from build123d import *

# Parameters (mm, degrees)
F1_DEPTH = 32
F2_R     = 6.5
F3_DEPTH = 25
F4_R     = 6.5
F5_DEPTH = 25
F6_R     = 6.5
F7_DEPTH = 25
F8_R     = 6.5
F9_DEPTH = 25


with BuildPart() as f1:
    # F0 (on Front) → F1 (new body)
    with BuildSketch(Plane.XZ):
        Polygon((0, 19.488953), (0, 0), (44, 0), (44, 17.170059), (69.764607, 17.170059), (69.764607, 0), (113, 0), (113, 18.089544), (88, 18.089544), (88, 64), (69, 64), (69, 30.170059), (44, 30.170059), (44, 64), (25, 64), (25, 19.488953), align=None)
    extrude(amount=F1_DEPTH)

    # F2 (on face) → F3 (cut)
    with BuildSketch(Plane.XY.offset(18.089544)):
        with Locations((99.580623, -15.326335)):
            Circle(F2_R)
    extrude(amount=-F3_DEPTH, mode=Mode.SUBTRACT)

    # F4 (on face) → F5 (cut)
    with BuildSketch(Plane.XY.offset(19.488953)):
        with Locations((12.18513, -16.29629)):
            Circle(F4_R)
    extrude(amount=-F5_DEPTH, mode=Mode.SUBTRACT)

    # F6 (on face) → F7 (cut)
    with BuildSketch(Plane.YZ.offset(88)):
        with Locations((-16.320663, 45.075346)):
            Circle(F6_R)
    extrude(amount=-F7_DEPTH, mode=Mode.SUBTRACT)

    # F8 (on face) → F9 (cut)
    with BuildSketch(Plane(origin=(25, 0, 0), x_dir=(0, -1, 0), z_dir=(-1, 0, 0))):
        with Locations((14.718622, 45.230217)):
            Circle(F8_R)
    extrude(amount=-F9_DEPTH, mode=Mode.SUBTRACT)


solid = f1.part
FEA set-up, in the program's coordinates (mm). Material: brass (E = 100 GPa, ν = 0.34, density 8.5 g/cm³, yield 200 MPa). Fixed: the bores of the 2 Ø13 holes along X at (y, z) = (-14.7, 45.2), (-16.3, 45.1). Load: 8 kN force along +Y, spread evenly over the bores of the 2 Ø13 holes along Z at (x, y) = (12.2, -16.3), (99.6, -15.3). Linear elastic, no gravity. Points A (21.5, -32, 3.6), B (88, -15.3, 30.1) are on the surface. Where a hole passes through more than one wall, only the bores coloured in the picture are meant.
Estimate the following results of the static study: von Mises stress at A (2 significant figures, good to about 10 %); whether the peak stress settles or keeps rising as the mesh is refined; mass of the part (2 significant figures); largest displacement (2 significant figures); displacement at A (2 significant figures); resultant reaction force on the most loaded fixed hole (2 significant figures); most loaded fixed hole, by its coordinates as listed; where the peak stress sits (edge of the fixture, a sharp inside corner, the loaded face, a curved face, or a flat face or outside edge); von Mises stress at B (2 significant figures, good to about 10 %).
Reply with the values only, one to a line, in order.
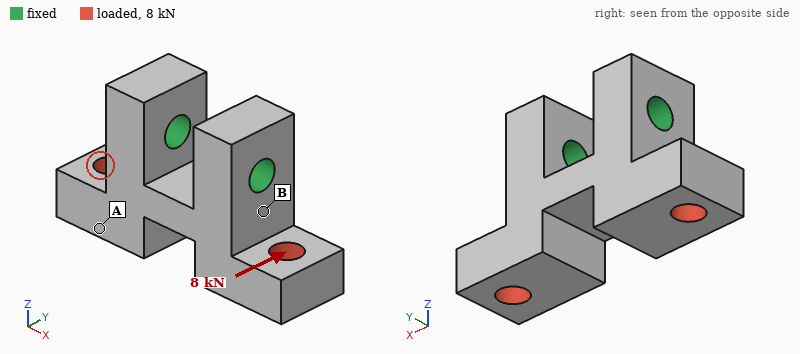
14 MPa
keeps rising
920 g
63 µm
41 µm
4.2 kN
(-14.7, 45.2)
edge of the fixture
36 MPa
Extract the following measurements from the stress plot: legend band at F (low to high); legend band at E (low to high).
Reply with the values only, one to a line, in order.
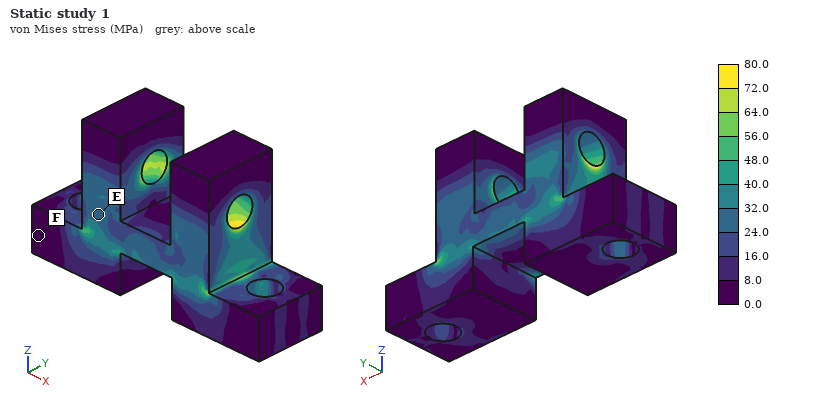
0.0 to 8.0 MPa
24.0 to 32.0 MPa
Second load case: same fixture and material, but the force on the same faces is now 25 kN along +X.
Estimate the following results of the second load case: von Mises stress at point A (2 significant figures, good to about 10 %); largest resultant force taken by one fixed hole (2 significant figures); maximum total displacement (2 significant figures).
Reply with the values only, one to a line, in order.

20 MPa
15 kN
0.10 mm
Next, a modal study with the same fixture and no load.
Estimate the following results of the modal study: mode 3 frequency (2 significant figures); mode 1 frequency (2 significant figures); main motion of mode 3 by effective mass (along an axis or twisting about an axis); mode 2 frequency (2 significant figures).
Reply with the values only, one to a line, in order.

4100 Hz
3800 Hz
along X
3800 Hz
